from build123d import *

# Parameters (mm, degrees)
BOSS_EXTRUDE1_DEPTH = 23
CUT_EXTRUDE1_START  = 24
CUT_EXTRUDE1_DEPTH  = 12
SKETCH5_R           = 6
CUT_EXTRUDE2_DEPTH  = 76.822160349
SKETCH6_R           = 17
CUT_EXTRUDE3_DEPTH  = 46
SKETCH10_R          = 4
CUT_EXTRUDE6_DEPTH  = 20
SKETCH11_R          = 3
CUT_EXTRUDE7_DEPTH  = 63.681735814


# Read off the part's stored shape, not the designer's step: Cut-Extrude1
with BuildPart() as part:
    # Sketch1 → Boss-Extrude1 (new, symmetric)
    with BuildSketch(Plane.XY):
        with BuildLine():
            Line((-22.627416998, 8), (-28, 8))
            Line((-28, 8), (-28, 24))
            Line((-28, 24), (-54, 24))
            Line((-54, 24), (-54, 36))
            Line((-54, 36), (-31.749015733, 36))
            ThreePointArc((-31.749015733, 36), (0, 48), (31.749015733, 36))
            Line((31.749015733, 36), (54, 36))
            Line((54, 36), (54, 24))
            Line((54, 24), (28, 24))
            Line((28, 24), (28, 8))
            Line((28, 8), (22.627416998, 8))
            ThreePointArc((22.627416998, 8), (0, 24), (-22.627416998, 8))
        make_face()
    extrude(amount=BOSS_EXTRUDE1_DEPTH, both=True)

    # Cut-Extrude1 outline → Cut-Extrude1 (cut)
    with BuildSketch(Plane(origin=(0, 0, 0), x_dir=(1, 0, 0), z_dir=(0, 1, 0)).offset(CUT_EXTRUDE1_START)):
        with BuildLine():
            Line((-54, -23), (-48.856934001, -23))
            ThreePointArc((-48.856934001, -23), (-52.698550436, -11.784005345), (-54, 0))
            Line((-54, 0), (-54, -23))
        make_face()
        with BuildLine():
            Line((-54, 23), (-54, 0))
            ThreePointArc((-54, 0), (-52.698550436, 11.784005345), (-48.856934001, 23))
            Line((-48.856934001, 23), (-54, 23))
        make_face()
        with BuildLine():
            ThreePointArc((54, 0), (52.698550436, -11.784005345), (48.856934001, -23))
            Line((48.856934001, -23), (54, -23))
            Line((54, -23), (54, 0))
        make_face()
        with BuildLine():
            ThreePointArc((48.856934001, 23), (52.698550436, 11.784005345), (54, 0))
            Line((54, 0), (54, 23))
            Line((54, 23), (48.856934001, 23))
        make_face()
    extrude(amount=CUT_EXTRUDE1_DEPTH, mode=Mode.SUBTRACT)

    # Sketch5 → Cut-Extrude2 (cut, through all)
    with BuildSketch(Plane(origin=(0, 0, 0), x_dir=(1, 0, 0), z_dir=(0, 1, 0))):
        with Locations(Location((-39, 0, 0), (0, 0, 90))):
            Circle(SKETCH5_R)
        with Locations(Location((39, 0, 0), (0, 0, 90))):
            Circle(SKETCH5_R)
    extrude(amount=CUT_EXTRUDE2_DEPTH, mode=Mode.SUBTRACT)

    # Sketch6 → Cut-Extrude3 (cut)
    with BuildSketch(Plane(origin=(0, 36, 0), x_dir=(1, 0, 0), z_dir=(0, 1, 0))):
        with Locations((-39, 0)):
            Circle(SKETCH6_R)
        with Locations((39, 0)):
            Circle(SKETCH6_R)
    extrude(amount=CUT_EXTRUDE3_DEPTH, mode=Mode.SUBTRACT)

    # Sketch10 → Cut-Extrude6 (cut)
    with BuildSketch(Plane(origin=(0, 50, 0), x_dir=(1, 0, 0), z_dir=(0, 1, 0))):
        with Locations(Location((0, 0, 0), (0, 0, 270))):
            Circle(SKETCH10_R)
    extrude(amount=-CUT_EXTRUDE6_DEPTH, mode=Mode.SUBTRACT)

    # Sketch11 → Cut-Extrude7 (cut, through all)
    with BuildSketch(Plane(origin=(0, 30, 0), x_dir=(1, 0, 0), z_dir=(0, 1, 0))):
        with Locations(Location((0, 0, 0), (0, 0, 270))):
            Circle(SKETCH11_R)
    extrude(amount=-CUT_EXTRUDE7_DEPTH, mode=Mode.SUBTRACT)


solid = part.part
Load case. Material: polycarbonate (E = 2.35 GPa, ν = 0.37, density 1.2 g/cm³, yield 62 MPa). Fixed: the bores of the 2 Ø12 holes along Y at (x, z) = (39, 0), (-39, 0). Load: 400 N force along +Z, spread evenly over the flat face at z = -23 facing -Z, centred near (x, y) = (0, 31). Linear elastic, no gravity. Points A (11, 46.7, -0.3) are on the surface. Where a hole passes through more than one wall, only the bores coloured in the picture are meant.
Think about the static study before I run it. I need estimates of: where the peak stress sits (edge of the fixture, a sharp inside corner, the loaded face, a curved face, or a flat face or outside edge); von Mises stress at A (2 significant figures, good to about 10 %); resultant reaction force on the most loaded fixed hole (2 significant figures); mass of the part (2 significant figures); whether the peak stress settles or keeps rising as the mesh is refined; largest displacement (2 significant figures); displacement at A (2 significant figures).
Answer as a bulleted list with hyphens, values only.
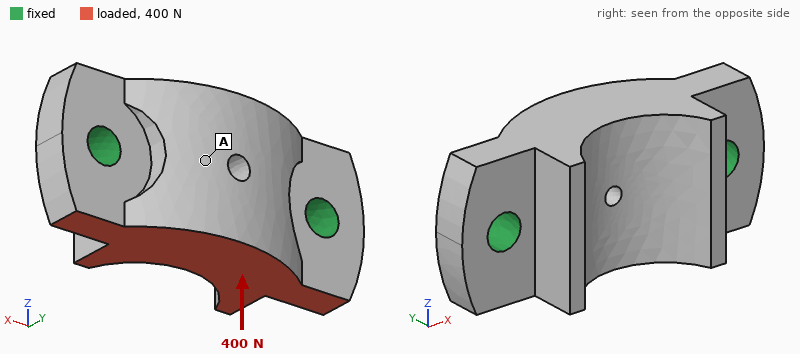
- edge of the fixture
- 0.23 MPa
- 200 N
- 110 g
- keeps rising
- 16 µm
- 12 µm
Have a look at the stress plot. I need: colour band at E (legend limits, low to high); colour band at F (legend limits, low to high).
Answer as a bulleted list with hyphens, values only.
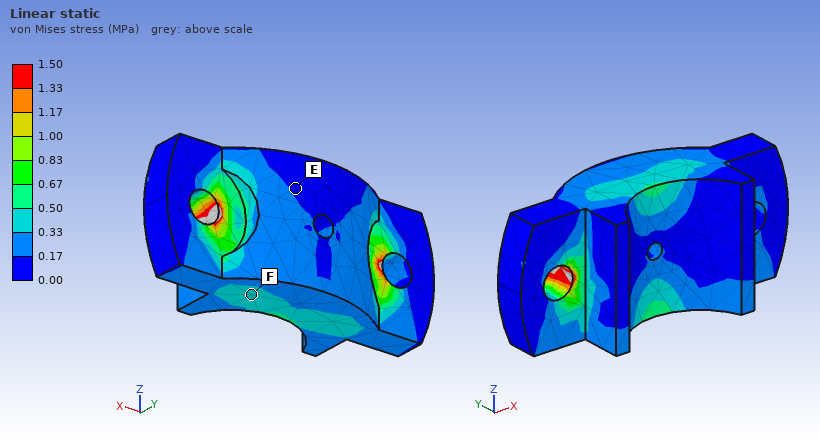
- 0.00 to 0.17 MPa
- 0.33 to 0.50 MPa
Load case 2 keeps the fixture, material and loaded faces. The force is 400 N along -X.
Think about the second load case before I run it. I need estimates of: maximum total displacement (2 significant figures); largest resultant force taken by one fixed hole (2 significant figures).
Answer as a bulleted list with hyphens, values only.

- 15 µm
- 230 N
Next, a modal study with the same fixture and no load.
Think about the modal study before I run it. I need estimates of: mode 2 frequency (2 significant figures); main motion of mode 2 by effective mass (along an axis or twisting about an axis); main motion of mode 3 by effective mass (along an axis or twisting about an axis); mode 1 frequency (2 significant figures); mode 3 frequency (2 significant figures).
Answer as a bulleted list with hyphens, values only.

- 2500 Hz
- along Y
- along Z
- 2000 Hz
- 3200 Hz
